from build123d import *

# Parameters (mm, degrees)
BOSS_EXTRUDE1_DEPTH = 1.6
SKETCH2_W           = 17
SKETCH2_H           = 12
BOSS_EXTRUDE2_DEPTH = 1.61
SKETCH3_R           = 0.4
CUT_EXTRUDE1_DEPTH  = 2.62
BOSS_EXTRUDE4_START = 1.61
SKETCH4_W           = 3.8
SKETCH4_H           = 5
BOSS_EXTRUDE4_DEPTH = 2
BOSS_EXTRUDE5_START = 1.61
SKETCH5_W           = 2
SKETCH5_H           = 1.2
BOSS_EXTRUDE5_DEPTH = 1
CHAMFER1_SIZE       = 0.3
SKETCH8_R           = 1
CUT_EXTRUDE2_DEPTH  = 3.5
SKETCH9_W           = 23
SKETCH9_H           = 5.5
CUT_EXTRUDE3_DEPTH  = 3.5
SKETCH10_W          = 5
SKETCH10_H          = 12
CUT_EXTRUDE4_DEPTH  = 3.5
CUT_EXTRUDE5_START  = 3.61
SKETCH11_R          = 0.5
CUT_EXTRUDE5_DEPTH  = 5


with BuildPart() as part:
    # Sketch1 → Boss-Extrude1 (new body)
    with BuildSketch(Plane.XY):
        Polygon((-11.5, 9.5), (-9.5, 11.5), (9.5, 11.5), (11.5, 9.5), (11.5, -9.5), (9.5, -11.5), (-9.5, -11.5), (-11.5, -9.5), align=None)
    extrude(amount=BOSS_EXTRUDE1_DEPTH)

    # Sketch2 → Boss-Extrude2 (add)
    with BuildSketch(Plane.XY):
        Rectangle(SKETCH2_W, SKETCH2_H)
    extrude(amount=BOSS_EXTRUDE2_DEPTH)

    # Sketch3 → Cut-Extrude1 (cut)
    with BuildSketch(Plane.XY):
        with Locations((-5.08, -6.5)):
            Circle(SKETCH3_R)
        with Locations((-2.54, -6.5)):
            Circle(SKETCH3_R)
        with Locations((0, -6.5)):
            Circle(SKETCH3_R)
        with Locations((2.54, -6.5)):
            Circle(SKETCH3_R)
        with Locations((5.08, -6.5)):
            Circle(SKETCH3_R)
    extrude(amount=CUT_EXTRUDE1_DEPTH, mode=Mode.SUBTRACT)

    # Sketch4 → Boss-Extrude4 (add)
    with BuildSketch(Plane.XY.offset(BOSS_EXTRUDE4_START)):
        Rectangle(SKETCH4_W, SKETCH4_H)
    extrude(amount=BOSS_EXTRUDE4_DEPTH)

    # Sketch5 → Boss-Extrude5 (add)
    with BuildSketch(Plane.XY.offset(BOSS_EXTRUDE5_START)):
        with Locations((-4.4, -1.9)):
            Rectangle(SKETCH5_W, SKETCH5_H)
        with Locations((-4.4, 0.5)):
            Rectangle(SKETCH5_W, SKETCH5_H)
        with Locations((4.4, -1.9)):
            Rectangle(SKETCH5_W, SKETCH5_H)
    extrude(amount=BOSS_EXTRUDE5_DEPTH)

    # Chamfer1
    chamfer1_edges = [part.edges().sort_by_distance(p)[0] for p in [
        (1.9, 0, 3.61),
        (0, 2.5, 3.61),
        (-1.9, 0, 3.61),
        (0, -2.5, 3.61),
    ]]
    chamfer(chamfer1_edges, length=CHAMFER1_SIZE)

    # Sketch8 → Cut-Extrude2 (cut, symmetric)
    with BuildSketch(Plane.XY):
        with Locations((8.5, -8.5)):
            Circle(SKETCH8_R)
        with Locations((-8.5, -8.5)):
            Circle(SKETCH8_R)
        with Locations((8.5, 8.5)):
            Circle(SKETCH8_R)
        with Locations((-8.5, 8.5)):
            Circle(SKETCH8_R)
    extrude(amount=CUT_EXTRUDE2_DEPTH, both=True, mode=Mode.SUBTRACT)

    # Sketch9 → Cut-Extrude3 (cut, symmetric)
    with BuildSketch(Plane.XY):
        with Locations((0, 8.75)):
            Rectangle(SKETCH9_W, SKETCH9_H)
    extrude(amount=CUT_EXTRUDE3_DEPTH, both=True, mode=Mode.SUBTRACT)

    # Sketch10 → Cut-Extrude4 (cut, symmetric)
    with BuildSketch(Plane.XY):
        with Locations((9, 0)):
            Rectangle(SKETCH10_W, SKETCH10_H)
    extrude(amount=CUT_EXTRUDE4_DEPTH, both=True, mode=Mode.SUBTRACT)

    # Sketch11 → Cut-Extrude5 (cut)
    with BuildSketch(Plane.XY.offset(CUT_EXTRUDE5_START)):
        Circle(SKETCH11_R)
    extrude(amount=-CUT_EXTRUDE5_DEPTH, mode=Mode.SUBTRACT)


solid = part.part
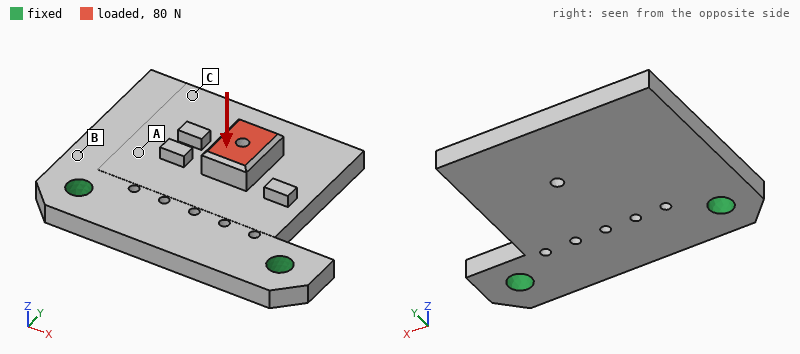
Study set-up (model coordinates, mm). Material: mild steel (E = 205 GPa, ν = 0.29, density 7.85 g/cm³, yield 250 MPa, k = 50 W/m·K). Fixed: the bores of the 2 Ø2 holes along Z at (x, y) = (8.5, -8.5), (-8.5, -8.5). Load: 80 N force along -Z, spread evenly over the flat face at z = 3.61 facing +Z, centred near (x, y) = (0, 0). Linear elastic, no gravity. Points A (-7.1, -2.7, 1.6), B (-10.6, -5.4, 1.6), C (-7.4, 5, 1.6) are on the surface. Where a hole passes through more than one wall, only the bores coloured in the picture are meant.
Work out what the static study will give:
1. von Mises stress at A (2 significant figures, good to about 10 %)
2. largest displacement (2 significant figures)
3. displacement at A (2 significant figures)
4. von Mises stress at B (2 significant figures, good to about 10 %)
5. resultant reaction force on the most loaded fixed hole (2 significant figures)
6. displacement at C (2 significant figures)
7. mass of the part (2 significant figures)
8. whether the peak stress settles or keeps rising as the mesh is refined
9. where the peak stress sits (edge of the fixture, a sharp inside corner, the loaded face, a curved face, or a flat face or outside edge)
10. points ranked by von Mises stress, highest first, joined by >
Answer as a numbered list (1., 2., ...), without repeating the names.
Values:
1. 35 MPa
2. 44 µm
3. 9.6 µm
4. 77 MPa
5. 41 N
6. 31 µm
7. 4.5 g
8. keeps rising
9. a sharp inside corner
10. B > A > C
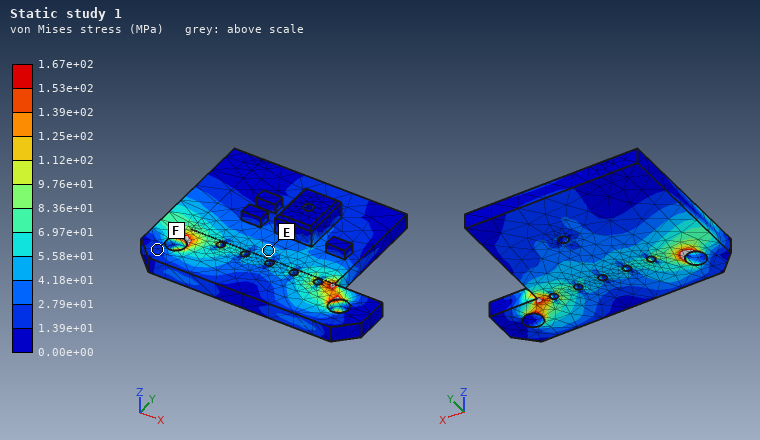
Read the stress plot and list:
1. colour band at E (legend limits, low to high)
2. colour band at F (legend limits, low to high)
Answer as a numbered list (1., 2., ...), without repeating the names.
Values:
1. 4.18e+01 to 5.58e+01 MPa
2. 1.39e+01 to 2.79e+01 MPa
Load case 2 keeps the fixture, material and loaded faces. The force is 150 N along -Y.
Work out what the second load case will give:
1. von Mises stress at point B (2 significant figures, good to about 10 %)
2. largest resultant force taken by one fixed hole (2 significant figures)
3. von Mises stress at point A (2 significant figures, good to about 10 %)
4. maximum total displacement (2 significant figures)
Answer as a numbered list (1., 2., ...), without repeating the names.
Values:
1. 61 MPa
2. 82 N
3. 45 MPa
4. 36 µm
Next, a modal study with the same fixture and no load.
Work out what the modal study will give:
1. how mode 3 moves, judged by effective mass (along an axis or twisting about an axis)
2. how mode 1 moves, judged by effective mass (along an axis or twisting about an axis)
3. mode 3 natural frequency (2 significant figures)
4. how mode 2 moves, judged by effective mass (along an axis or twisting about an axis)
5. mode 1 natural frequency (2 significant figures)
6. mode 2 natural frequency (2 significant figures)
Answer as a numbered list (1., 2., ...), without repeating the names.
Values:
1. along Z
2. along Z
3. 27 kHz
4. twisting about Y
5. 5200 Hz
6. 14 kHz
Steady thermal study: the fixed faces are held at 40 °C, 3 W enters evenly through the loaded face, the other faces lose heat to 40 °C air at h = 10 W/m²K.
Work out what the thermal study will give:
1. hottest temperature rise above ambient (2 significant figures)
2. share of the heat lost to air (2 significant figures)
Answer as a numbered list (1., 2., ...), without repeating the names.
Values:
1. 35 K
2. 4.2 %
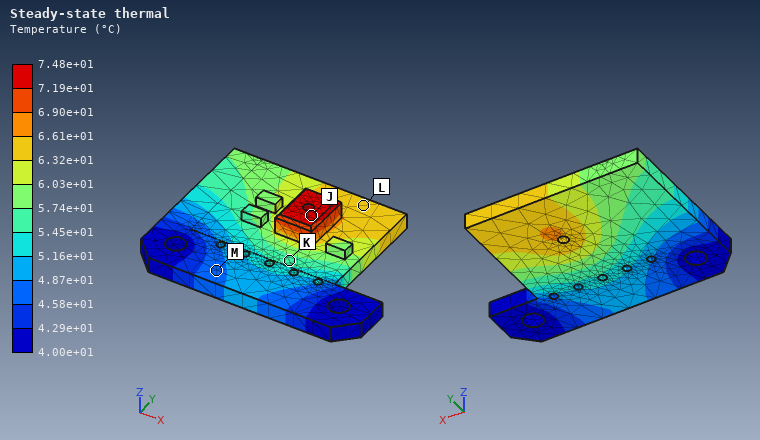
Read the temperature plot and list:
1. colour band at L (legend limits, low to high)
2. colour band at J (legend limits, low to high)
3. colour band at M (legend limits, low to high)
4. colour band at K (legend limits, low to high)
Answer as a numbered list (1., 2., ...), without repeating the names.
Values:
1. 6.32e+01 to 6.61e+01 °C
2. 7.19e+01 to 7.48e+01 °C
3. 4.58e+01 to 4.87e+01 °C
4. 5.45e+01 to 5.74e+01 °C
